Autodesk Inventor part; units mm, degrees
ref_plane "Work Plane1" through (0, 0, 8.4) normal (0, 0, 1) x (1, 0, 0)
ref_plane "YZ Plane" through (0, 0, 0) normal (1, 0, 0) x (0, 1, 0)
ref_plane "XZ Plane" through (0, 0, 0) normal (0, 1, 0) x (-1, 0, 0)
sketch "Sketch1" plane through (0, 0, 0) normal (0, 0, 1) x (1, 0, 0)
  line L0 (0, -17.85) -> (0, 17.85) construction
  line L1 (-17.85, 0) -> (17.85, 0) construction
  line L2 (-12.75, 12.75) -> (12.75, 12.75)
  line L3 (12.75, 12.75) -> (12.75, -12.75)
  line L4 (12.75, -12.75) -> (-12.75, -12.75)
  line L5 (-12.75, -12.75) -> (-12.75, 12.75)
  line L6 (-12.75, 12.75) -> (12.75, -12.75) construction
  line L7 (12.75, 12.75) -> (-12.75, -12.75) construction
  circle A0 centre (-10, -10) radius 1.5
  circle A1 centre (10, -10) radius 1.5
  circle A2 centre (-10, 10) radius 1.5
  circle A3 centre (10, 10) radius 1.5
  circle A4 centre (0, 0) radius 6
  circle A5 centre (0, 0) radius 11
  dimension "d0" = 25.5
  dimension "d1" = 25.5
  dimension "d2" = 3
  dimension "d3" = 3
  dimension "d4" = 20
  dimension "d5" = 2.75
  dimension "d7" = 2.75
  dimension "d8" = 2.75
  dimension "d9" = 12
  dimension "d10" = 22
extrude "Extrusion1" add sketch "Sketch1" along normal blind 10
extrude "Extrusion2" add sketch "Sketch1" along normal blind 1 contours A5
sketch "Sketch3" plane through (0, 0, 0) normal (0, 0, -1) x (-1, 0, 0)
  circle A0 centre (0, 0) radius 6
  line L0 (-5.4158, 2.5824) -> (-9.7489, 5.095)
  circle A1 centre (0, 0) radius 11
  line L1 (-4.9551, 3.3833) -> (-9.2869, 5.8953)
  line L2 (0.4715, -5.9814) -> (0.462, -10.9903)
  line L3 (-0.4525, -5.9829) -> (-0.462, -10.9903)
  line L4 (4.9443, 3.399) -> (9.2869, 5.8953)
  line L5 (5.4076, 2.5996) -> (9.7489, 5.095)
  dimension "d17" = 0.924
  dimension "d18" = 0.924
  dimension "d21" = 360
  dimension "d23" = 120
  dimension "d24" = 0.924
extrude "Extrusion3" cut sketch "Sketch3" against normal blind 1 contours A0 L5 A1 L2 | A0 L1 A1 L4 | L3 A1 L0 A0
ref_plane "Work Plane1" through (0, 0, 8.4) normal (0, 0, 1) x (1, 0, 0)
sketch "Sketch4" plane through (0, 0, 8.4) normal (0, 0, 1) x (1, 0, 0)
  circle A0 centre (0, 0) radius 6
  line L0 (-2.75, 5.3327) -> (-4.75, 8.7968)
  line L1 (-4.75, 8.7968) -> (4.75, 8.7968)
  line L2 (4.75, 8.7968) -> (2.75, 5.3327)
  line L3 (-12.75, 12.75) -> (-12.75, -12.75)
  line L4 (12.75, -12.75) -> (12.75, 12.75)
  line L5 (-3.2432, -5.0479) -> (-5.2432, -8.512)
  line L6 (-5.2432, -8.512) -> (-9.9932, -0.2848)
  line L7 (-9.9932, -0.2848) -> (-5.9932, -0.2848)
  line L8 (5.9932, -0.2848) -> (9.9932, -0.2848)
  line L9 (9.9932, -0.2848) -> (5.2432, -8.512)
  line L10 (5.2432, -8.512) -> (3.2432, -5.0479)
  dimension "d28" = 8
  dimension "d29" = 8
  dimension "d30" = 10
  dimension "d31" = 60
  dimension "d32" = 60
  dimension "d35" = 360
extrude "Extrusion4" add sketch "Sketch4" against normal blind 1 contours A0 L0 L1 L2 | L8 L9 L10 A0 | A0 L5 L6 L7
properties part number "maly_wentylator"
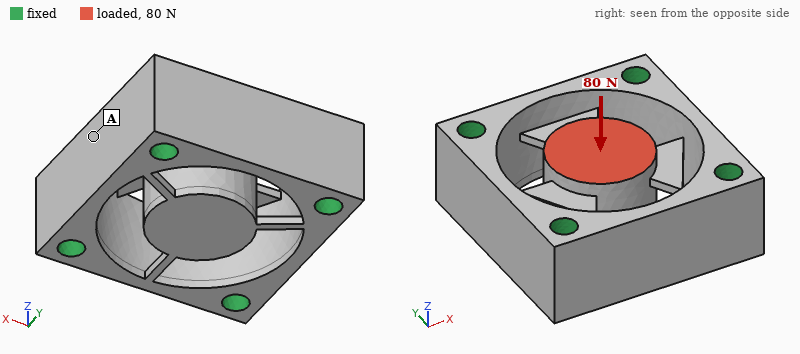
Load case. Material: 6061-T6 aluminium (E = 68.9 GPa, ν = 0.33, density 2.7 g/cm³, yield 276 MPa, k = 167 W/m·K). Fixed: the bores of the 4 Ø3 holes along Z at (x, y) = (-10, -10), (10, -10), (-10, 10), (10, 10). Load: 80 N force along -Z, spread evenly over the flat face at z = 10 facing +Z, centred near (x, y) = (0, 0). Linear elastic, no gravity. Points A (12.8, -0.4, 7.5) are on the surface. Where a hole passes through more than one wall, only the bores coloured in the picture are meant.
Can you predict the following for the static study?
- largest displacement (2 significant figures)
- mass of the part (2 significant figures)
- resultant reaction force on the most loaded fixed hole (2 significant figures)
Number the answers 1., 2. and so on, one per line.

1. 81 µm
2. 9.8 g
3. 24 N
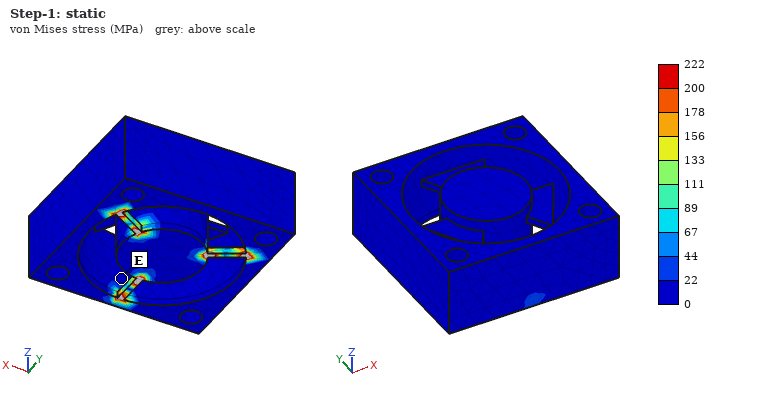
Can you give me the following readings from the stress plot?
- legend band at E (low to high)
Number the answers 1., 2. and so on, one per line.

1. 0 to 22 MPa
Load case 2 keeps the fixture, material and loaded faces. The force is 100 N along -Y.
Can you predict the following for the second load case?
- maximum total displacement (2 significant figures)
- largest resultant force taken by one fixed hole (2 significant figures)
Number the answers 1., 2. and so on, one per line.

1. 0.30 mm
2. 57 N
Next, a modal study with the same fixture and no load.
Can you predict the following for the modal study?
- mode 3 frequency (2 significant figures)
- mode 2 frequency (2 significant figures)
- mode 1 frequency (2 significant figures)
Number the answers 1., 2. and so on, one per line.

1. 2800 Hz
2. 2700 Hz
3. 2700 Hz
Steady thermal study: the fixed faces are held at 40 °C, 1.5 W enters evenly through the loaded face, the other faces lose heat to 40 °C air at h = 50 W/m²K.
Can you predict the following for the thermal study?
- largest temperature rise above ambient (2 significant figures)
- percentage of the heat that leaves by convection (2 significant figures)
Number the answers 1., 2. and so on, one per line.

1. 14 K
2. 32 %
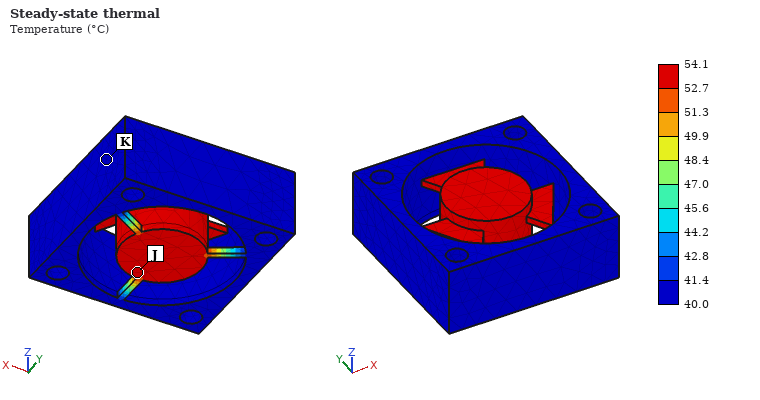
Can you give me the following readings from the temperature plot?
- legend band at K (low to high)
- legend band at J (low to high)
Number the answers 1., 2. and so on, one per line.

1. 40.0 to 41.4 °C
2. 52.7 to 54.1 °C
